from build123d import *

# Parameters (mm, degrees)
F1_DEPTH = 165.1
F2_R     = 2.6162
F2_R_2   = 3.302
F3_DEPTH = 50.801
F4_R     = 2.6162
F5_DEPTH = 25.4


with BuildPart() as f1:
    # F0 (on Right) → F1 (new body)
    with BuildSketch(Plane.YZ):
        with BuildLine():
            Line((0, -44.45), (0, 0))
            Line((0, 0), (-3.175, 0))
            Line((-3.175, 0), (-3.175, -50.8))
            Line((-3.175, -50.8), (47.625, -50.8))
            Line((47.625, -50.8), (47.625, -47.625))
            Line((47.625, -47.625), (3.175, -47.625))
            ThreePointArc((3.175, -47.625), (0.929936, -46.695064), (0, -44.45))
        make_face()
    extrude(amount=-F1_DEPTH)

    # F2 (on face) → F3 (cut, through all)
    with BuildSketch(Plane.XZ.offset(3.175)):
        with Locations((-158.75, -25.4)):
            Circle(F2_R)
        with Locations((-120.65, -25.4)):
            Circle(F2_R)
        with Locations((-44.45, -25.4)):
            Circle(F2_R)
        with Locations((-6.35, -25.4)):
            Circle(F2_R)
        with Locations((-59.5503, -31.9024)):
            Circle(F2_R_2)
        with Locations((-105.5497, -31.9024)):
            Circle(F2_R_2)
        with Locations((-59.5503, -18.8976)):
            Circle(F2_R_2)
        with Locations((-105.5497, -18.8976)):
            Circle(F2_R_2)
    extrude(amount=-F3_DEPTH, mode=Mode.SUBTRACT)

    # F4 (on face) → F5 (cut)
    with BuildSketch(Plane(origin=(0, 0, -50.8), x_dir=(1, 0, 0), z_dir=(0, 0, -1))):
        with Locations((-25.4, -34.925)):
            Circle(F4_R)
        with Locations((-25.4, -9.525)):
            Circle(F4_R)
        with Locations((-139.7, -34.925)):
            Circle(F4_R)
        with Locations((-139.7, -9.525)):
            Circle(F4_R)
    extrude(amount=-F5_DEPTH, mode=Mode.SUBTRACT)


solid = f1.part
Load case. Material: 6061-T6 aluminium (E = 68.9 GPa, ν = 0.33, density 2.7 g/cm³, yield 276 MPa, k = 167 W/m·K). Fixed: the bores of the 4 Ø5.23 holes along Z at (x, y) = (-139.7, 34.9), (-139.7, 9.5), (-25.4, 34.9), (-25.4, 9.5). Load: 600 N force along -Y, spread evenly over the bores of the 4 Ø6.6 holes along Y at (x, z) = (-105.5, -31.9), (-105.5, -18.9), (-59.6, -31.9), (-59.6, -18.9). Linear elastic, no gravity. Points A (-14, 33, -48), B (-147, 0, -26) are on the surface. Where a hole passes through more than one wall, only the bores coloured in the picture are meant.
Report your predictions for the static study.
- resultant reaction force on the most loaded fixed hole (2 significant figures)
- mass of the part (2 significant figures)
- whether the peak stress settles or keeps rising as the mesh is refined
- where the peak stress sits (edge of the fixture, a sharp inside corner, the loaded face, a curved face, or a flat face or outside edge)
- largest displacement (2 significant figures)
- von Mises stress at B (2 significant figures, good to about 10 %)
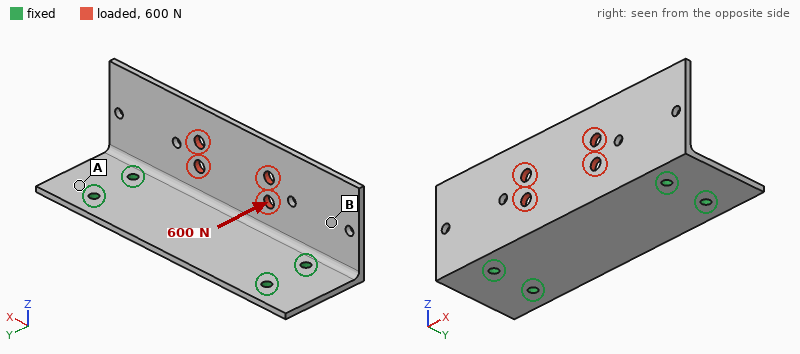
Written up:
300 N
140 g
keeps rising
edge of the fixture
0.64 mm
19 MPa
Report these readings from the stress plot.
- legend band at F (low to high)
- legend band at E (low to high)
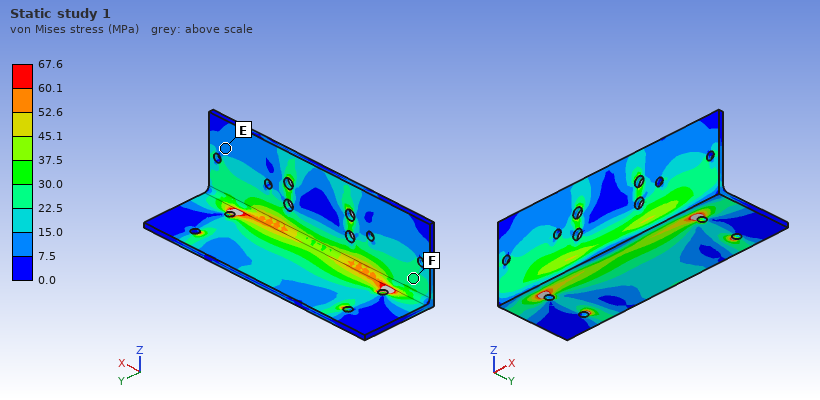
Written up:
22.5 to 30.0 MPa
7.5 to 15.0 MPa
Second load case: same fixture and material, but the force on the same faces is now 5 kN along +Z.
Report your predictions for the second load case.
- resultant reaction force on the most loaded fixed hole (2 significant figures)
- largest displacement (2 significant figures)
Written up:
3.4 kN
0.78 mm
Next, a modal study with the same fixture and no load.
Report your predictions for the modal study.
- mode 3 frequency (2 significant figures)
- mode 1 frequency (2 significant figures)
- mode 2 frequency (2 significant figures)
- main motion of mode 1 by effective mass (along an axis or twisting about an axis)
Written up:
1600 Hz
770 Hz
1100 Hz
along Y
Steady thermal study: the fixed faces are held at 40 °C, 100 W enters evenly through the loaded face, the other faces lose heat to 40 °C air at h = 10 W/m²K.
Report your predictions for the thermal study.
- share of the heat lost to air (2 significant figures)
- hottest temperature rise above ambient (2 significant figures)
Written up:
11 %
83 K
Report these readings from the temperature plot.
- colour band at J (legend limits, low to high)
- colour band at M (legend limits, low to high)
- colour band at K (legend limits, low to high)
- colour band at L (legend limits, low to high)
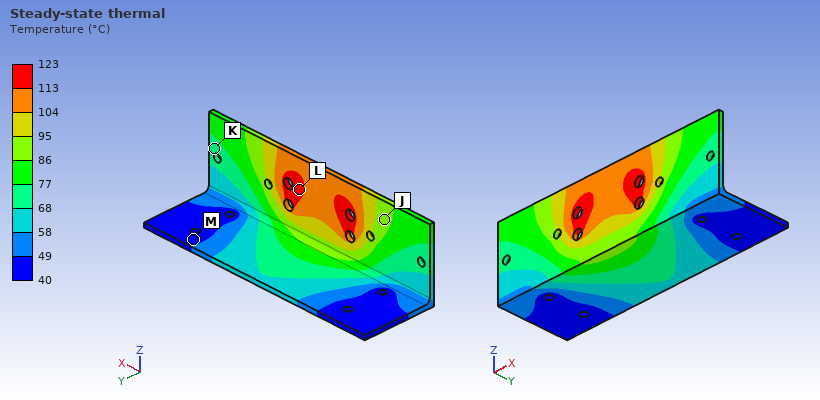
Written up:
86 to 95 °C
40 to 49 °C
68 to 77 °C
113 to 123 °C
